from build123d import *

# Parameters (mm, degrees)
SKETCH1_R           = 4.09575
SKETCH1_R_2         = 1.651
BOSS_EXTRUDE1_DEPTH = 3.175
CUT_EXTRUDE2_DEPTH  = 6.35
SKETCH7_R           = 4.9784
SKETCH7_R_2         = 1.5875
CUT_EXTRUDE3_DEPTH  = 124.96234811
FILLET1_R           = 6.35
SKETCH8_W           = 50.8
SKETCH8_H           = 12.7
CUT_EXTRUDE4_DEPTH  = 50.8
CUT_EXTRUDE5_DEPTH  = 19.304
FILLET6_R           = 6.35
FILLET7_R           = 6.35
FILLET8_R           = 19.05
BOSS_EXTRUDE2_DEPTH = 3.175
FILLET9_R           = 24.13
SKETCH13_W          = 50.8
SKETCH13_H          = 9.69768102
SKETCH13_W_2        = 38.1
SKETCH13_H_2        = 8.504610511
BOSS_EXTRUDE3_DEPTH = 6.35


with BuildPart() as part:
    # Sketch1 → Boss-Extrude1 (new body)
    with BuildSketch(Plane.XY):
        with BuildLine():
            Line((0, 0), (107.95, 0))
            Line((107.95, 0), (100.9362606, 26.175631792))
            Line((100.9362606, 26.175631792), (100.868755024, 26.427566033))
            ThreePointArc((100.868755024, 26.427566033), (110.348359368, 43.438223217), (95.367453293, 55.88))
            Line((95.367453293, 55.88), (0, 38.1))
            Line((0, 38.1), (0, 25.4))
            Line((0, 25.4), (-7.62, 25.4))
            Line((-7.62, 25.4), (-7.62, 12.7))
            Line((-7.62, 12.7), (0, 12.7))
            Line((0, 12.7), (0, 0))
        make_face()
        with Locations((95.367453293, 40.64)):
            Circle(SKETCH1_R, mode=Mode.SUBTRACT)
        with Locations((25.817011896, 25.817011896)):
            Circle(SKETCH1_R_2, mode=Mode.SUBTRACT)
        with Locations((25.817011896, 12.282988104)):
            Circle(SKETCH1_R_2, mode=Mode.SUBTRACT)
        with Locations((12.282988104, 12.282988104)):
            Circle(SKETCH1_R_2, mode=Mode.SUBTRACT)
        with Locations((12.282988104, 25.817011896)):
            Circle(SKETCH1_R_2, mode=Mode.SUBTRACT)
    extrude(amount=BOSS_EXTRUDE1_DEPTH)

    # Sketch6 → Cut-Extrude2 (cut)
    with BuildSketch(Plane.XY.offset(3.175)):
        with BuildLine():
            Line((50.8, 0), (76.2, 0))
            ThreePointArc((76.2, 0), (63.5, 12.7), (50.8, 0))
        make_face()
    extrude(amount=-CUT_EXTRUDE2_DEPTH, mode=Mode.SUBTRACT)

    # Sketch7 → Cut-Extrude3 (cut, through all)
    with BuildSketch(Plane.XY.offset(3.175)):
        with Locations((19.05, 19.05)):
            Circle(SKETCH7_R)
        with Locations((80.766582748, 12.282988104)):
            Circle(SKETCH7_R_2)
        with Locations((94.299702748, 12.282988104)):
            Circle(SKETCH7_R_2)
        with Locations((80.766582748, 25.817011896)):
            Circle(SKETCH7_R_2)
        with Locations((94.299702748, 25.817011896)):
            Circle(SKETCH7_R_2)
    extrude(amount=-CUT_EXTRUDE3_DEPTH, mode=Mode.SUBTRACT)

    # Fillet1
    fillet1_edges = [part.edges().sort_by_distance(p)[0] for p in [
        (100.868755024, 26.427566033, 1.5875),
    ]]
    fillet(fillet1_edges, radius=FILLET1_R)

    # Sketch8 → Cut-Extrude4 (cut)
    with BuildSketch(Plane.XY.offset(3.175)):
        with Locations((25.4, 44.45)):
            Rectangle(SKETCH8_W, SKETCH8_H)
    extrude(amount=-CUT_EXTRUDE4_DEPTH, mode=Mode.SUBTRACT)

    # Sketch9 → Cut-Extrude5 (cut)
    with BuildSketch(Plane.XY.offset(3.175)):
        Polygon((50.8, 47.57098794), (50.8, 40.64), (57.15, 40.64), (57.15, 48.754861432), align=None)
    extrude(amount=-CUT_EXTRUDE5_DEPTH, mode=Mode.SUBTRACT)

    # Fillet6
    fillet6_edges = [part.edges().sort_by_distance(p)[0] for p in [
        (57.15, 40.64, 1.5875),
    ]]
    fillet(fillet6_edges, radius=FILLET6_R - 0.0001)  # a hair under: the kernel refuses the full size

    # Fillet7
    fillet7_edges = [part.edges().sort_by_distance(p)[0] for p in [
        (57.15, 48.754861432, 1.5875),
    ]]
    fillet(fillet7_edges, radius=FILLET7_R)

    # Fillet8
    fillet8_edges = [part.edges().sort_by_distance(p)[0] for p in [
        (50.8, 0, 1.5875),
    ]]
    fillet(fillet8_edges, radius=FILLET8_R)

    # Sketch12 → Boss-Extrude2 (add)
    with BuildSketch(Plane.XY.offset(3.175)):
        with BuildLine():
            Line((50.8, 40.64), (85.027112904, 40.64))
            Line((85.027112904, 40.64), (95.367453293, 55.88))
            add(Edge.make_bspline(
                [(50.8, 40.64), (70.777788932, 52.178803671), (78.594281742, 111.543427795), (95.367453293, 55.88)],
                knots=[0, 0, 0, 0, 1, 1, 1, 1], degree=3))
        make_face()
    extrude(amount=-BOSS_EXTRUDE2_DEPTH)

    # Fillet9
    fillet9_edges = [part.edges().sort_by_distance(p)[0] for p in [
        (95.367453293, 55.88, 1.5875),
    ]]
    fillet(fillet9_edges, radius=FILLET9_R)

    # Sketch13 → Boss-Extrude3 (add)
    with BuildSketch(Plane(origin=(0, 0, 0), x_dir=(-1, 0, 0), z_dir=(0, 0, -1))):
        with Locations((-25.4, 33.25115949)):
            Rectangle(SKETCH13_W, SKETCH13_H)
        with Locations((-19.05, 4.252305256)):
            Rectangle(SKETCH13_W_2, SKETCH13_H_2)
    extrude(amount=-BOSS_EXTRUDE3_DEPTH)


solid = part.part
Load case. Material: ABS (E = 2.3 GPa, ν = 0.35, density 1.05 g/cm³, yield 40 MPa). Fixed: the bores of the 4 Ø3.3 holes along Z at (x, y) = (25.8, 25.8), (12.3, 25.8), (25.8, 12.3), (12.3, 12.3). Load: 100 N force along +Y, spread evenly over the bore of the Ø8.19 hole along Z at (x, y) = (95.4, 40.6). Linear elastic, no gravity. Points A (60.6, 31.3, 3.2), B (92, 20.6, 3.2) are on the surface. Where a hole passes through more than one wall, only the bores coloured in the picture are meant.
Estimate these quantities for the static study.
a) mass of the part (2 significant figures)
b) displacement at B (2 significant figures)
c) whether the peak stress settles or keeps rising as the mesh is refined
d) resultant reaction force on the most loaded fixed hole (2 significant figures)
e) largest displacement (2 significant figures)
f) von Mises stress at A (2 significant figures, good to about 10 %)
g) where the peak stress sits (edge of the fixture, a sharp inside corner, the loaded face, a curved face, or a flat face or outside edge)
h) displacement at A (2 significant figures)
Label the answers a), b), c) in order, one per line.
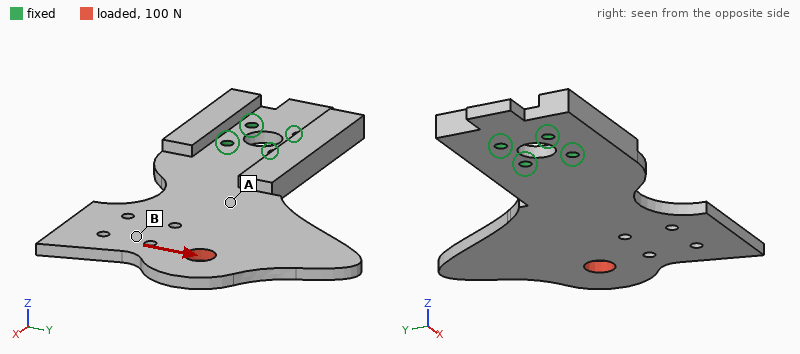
a) 19 g
b) 0.74 mm
c) keeps rising
d) 250 N
e) 1.2 mm
f) 4.1 MPa
g) edge of the fixture
h) 0.33 mm
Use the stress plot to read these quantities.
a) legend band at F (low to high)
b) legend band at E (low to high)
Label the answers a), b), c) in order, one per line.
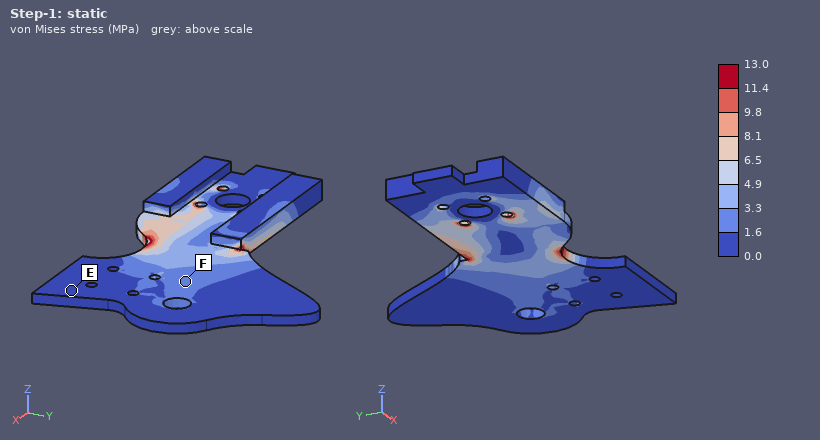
a) 1.6 to 3.3 MPa
b) 0.0 to 1.6 MPa
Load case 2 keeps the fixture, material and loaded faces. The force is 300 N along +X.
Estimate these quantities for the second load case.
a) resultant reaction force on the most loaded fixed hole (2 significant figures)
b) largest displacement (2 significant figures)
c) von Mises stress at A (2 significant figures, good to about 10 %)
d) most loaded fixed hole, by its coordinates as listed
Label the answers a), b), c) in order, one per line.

a) 320 N
b) 1.5 mm
c) 6.1 MPa
d) (25.8, 25.8)
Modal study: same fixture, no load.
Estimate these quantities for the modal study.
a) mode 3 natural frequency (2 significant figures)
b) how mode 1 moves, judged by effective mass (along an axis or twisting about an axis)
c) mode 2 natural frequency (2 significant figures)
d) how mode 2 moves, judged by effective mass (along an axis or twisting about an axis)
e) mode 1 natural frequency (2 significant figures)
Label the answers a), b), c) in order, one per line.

a) 690 Hz
b) along Z
c) 250 Hz
d) twisting about X
e) 120 Hz
